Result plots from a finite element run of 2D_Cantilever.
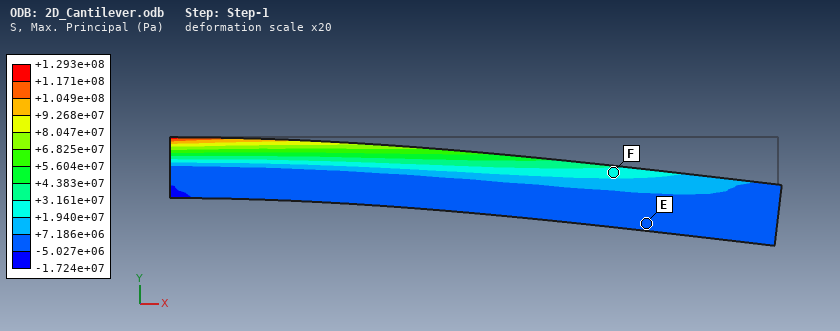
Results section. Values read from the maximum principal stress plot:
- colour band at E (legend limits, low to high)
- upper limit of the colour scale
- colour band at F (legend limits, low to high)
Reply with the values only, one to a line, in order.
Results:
-5.027e+06 to +7.186e+06 Pa
+1.293e+08 Pa
+1.940e+07 to +3.161e+07 Pa
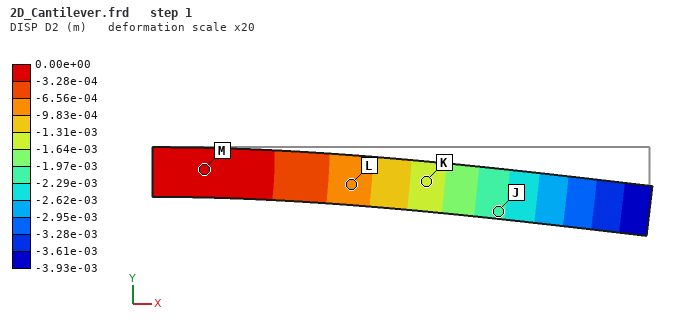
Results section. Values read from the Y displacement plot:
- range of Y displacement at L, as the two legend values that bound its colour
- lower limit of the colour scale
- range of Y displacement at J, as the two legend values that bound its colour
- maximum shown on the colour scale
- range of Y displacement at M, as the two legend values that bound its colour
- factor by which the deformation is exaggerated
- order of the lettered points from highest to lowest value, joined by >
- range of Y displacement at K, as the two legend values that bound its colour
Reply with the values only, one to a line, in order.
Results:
-9.83e-04 to -6.56e-04 m
-3.93e-03 m
-2.29e-03 to -1.97e-03 m
0.00e+00 m
-3.28e-04 to 0.00e+00 m
20
M > L > K > J
-1.64e-03 to -1.31e-03 m
